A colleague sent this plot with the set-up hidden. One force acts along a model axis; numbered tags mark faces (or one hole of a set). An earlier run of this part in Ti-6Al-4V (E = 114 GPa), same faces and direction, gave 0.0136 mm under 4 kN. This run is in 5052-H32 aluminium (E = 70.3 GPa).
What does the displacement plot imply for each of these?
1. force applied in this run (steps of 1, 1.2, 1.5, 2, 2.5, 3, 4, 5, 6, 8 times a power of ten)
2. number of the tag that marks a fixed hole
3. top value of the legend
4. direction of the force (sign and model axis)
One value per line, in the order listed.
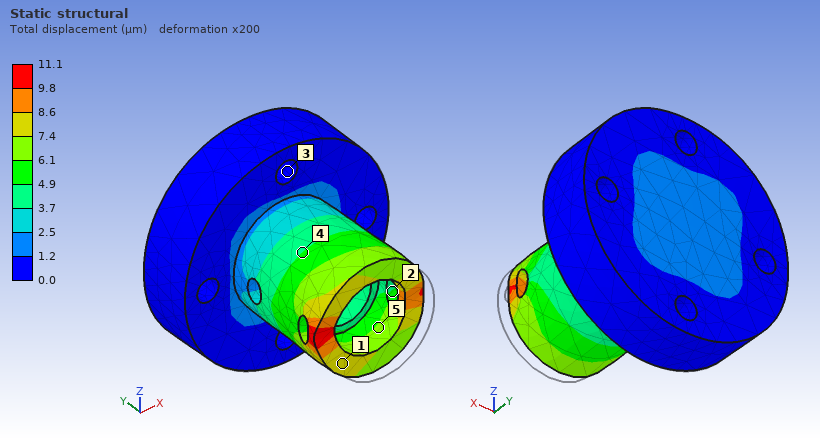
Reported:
2 kN
3
11.1 µm
+Y
